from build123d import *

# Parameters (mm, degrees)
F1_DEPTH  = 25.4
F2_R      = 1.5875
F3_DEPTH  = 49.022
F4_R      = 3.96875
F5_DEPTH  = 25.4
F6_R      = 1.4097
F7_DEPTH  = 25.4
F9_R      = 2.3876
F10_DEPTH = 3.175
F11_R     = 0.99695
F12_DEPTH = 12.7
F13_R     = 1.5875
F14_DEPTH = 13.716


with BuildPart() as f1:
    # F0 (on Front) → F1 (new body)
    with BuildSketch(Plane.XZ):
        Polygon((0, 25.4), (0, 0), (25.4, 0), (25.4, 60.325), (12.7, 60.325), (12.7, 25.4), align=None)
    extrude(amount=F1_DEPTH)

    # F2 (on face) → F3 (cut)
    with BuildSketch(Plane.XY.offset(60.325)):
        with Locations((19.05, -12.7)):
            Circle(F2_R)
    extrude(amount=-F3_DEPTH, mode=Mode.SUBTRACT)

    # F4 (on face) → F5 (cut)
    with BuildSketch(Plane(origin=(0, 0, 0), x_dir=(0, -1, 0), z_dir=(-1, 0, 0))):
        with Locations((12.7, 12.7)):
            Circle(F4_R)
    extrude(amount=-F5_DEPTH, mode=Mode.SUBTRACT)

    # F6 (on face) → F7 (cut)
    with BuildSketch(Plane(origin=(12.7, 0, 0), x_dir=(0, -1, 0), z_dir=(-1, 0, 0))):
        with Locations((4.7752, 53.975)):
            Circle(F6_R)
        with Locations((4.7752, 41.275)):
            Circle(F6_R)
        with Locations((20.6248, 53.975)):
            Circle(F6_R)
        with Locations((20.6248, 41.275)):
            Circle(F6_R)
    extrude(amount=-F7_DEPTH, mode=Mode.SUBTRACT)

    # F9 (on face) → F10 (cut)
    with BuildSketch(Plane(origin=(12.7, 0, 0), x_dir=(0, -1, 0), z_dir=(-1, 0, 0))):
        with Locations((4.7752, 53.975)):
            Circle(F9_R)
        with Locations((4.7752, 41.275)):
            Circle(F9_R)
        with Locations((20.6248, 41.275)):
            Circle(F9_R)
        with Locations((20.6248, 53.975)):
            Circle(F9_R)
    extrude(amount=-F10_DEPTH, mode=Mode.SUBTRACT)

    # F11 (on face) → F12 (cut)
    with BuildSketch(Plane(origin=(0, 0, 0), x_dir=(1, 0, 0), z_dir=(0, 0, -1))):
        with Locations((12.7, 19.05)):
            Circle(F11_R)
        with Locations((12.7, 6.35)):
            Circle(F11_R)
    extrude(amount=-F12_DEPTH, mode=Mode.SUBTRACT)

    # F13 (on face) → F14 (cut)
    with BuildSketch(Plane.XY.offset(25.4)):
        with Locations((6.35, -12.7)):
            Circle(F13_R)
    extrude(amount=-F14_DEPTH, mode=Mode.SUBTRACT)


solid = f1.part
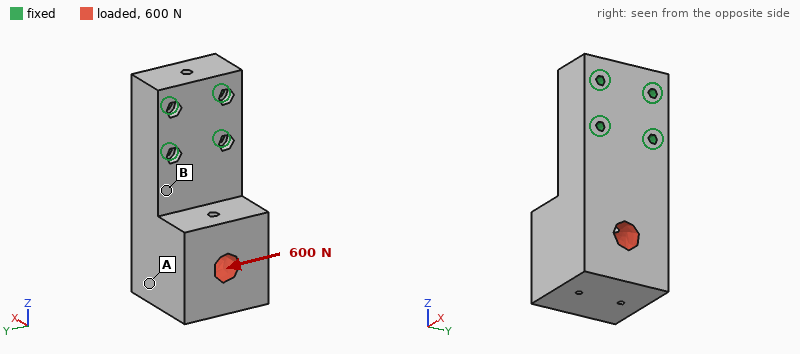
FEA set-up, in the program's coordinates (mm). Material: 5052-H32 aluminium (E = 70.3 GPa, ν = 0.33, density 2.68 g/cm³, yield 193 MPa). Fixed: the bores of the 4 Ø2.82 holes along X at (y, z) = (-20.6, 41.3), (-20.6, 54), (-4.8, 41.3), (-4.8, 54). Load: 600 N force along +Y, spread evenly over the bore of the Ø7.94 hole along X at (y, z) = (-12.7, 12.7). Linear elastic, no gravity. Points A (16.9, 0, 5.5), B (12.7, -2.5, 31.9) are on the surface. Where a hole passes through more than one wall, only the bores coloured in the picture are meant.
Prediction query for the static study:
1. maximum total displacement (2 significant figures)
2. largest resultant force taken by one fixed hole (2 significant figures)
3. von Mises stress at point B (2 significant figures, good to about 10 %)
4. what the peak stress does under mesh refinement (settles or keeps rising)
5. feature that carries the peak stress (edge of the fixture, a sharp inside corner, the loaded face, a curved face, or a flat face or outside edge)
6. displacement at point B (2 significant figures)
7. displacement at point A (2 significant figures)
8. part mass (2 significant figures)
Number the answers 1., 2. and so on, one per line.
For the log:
1. 13 µm
2. 910 N
3. 7.4 MPa
4. keeps rising
5. edge of the fixture
6. 2.7 µm
7. 9.7 µm
8. 68 g
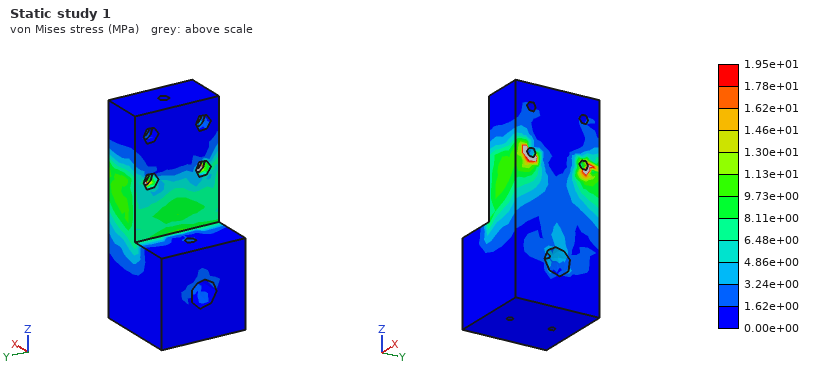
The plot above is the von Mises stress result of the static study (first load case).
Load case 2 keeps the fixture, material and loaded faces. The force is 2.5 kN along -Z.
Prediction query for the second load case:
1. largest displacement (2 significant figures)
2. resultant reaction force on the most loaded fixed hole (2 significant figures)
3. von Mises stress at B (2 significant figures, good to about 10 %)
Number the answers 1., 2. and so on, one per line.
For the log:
1. 54 µm
2. 920 N
3. 29 MPa
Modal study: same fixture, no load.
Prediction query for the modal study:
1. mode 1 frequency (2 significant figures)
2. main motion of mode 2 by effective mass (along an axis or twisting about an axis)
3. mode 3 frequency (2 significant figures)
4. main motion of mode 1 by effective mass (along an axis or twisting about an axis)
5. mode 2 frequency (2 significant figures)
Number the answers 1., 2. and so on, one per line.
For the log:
1. 3500 Hz
2. along Y
3. 9800 Hz
4. along X
5. 6400 Hz
